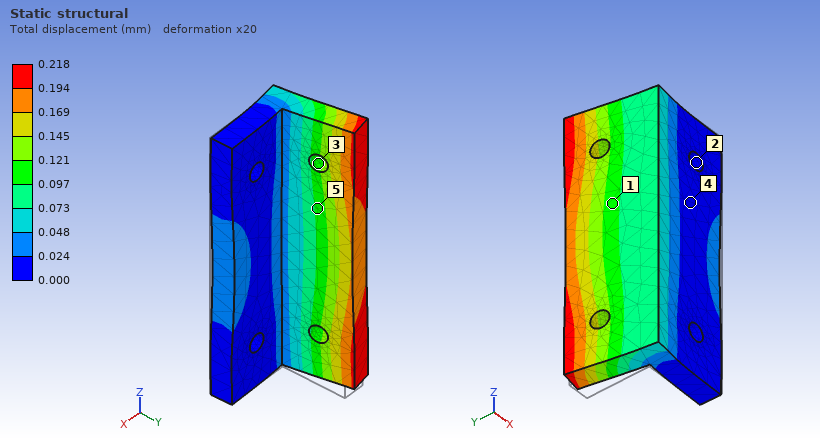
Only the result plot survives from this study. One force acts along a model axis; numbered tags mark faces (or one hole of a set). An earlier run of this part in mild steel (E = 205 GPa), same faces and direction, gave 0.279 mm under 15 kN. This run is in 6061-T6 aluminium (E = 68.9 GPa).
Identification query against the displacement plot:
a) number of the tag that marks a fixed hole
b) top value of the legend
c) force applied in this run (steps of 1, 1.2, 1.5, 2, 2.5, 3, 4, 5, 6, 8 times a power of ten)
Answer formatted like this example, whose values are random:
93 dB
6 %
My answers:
2
0.218 mm
4 kN
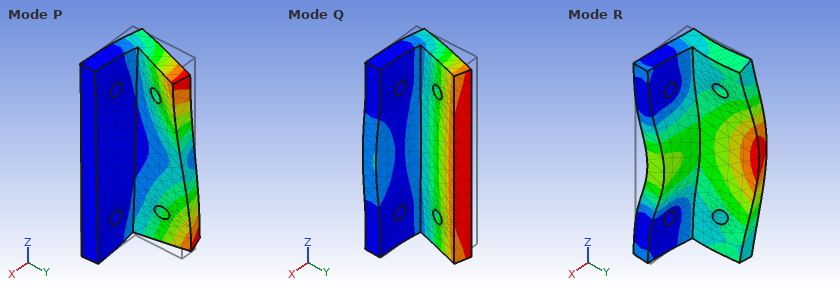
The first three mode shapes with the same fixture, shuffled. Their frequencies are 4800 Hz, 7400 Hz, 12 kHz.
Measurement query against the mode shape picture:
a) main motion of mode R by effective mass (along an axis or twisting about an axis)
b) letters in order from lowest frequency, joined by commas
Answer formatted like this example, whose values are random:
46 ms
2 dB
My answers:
along Y
Q, P, R
